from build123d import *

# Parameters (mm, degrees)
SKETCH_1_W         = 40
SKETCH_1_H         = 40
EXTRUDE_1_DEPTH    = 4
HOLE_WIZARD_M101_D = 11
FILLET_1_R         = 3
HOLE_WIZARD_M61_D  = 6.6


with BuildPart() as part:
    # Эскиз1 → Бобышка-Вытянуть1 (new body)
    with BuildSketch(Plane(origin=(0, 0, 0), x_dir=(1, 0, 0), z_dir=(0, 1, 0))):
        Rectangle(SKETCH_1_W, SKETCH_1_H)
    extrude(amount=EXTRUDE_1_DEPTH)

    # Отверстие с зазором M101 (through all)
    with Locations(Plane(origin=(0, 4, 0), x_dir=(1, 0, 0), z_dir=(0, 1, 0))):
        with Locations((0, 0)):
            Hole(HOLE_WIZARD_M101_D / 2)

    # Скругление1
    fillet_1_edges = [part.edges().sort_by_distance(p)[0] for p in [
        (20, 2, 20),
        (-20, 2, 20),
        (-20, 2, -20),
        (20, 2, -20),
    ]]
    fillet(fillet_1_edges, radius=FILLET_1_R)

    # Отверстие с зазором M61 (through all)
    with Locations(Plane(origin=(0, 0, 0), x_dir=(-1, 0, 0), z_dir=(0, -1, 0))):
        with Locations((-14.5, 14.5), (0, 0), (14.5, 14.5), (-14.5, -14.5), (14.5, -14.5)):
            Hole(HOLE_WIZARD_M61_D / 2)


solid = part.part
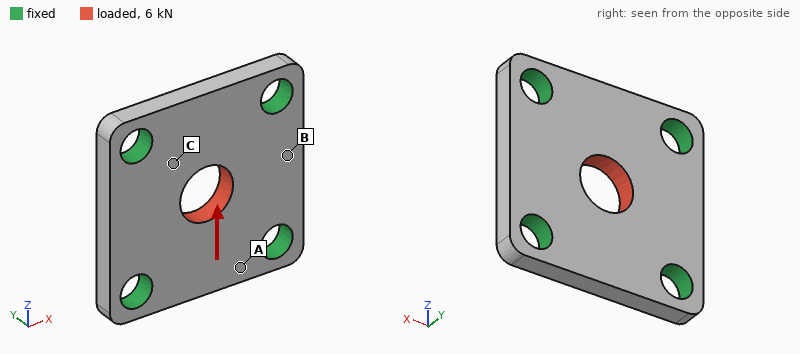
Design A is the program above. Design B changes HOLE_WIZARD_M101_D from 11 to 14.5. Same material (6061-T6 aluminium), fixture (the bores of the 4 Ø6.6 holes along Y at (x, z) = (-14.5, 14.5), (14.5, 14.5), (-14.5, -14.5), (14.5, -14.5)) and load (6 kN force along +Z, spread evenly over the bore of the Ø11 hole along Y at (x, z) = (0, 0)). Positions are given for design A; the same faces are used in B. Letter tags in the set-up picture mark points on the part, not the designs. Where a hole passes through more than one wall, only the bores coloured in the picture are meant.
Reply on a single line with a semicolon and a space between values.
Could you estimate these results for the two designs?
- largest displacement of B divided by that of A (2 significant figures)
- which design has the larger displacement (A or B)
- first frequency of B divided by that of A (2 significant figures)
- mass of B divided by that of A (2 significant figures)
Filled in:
0.91; A; 1.1; 0.95
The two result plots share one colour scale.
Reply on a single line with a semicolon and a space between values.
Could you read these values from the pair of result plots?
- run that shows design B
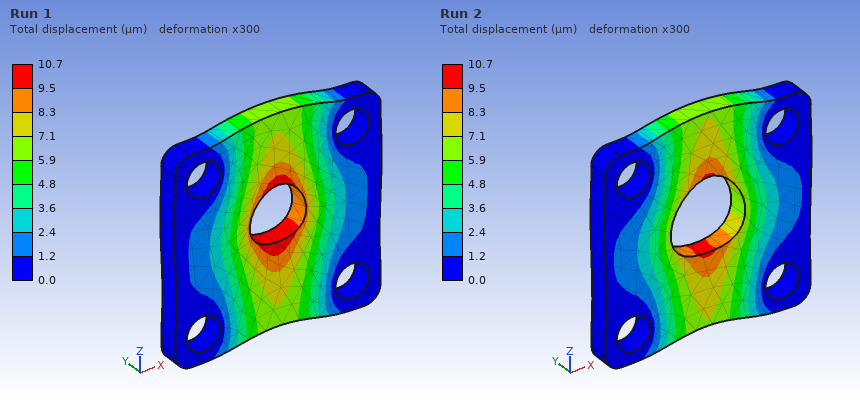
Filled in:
Run 2
